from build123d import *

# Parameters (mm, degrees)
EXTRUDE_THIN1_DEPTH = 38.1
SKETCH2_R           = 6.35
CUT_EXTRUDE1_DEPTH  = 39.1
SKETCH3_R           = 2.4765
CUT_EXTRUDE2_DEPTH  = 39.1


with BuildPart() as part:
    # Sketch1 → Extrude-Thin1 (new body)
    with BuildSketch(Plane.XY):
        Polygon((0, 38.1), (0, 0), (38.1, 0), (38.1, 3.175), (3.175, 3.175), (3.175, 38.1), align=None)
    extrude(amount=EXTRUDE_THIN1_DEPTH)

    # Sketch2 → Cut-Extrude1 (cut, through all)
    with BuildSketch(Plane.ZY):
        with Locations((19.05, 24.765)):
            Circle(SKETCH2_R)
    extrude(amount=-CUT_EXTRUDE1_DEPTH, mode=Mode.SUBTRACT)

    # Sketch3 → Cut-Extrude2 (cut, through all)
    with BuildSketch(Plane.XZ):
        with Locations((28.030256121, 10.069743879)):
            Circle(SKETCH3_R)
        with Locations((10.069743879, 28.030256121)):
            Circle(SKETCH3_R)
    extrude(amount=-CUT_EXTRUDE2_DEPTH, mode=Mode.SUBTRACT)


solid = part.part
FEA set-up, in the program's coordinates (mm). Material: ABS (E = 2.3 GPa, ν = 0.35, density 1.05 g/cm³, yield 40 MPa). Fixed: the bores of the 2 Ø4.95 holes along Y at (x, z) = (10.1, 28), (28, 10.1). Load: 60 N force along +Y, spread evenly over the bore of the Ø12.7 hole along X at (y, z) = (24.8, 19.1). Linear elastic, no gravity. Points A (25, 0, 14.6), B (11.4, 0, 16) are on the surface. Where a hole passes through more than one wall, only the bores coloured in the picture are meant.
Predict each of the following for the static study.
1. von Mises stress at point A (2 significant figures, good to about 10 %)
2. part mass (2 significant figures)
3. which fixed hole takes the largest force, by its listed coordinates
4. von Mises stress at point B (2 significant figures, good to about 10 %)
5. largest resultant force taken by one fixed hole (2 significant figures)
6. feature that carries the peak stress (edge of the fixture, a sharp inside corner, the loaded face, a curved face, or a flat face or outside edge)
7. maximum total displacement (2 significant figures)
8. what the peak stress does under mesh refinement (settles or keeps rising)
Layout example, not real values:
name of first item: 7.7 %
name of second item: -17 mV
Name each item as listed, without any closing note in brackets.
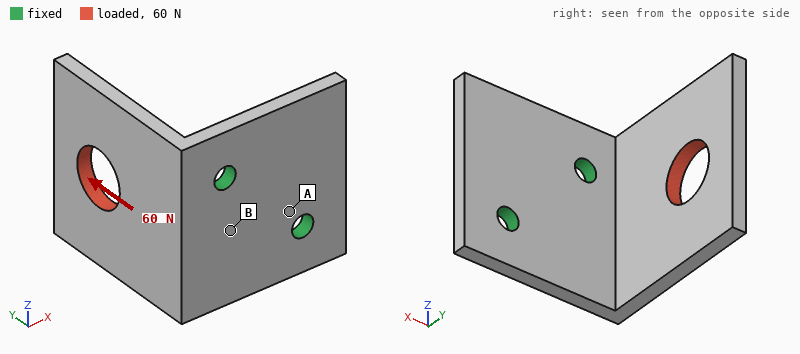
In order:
von Mises stress at point A: 1.9 MPa
part mass: 8.7 g
which fixed hole takes the largest force, by its listed coordinates: (10.1, 28)
von Mises stress at point B: 4.1 MPa
largest resultant force taken by one fixed hole: 56 N
feature that carries the peak stress: edge of the fixture
maximum total displacement: 0.77 mm
what the peak stress does under mesh refinement: keeps rising
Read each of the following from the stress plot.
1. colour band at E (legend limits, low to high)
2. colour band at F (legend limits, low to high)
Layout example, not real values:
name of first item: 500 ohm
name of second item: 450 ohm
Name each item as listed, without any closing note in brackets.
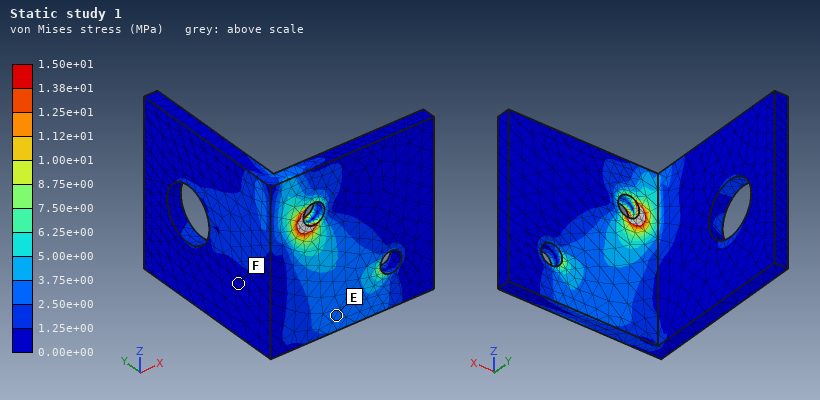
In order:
colour band at E: 2.50e+00 to 3.75e+00 MPa
colour band at F: 0.00e+00 to 1.25e+00 MPa
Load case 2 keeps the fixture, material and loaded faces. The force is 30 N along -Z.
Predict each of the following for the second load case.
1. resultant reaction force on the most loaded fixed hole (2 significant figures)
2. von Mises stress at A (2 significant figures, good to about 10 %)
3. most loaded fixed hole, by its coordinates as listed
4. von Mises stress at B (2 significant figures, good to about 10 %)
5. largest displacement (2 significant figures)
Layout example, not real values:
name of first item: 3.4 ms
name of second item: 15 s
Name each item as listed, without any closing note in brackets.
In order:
resultant reaction force on the most loaded fixed hole: 33 N
von Mises stress at A: 2.2 MPa
most loaded fixed hole, by its coordinates as listed: (10.1, 28)
von Mises stress at B: 3.4 MPa
largest displacement: 0.70 mm
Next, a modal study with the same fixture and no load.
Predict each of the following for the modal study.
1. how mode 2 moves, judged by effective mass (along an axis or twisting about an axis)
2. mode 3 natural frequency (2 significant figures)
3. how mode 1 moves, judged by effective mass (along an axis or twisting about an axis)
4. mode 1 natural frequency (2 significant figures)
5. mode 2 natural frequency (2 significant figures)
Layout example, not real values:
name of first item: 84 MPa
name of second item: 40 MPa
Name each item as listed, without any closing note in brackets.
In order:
how mode 2 moves, judged by effective mass: along Z
mode 3 natural frequency: 1200 Hz
how mode 1 moves, judged by effective mass: along X
mode 1 natural frequency: 420 Hz
mode 2 natural frequency: 710 Hz
